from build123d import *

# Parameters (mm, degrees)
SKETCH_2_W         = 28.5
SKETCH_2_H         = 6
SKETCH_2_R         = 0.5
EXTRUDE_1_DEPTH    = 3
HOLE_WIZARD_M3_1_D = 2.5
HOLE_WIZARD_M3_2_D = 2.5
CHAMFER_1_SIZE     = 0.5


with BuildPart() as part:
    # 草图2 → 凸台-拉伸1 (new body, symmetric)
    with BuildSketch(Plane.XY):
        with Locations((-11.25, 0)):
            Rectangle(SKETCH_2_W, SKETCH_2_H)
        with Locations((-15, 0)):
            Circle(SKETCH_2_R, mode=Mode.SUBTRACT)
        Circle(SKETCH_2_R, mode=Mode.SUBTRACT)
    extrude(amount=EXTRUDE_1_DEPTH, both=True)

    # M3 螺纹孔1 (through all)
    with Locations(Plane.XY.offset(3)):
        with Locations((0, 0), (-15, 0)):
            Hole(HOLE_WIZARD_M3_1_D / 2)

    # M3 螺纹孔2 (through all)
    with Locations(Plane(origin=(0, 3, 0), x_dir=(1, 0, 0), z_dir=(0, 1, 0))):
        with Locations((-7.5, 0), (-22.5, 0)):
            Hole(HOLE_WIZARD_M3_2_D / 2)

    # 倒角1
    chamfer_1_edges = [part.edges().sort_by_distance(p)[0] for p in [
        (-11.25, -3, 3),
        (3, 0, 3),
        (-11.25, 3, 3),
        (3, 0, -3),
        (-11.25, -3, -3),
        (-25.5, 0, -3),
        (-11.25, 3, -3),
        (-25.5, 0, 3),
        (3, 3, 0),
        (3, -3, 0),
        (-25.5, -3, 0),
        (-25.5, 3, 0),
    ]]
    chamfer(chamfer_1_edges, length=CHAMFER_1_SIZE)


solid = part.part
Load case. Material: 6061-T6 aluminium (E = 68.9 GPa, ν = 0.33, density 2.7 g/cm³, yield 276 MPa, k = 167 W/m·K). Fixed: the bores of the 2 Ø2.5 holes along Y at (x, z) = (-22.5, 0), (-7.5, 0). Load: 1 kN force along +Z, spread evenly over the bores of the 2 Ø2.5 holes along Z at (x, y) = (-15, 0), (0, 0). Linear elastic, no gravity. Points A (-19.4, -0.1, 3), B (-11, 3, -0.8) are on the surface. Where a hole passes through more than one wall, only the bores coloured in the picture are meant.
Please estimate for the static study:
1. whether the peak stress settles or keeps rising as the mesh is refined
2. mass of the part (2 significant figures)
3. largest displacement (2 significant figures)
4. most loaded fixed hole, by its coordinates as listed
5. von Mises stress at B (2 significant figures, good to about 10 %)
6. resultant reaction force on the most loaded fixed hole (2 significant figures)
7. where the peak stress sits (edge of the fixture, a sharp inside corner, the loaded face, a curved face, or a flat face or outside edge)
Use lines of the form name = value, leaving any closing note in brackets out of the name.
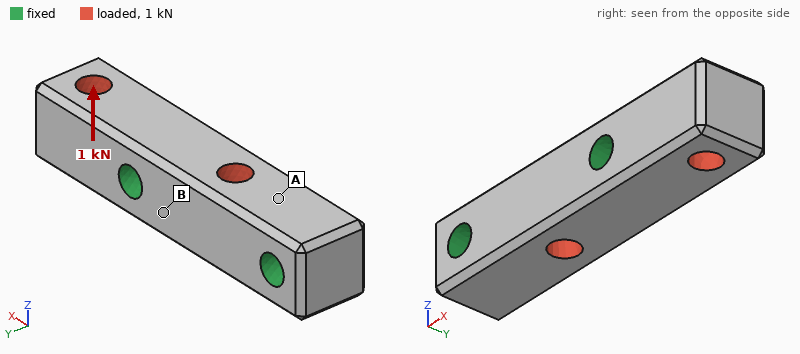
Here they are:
whether the peak stress settles or keeps rising as the mesh is refined = keeps rising
mass of the part = 2.4 g
largest displacement = 25 µm
most loaded fixed hole, by its coordinates as listed = (-7.5, 0)
von Mises stress at B = 22 MPa
resultant reaction force on the most loaded fixed hole = 810 N
where the peak stress sits = edge of the fixture
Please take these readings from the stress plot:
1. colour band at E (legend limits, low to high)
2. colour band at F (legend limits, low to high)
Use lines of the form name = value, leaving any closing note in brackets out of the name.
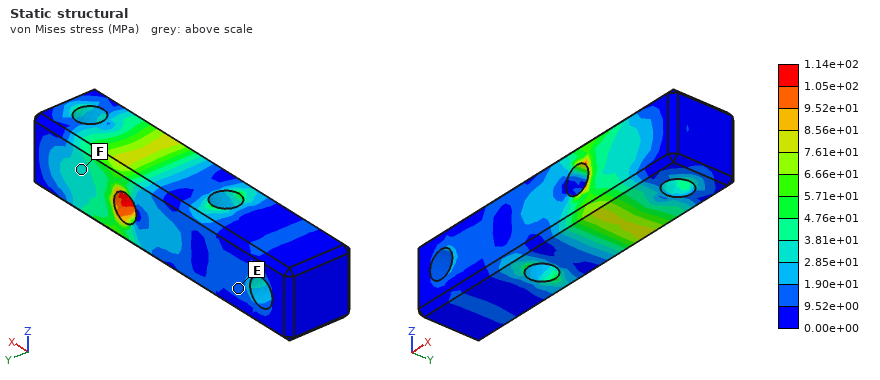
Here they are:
colour band at E = 9.52e+00 to 1.90e+01 MPa
colour band at F = 2.85e+01 to 3.81e+01 MPa
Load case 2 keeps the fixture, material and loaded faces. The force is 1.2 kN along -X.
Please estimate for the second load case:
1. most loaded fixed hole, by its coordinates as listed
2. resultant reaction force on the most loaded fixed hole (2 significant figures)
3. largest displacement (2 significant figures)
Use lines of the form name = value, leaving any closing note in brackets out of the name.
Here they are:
most loaded fixed hole, by its coordinates as listed = (-7.5, 0)
resultant reaction force on the most loaded fixed hole = 890 N
largest displacement = 3.0 µm
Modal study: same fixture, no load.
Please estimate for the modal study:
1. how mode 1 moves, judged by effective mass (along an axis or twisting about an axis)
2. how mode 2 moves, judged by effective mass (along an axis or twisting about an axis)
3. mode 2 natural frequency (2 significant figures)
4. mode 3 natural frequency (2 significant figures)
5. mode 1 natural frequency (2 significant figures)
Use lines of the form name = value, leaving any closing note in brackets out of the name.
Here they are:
how mode 1 moves, judged by effective mass = along Z
how mode 2 moves, judged by effective mass = along Y
mode 2 natural frequency = 40 kHz
mode 3 natural frequency = 73 kHz
mode 1 natural frequency = 35 kHz
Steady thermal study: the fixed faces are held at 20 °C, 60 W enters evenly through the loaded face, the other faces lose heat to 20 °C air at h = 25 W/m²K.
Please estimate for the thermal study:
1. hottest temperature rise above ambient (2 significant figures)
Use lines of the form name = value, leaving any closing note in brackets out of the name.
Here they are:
hottest temperature rise above ambient = 43 K
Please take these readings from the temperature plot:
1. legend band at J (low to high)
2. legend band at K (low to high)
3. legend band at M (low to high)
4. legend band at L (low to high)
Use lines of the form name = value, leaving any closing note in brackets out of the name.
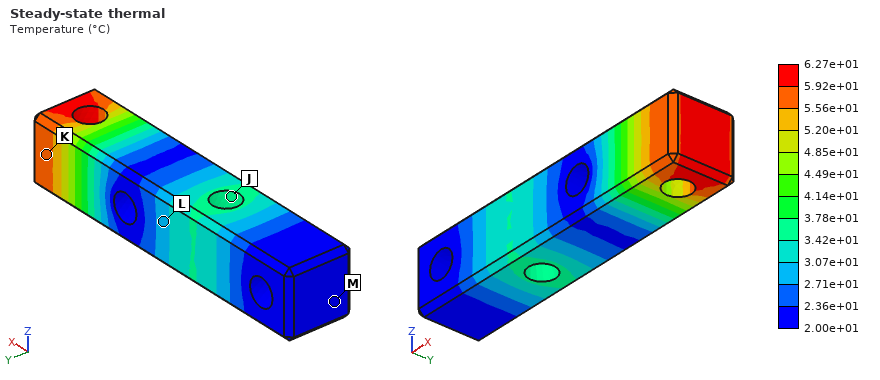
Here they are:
legend band at J = 3.42e+01 to 3.78e+01 °C
legend band at K = 5.56e+01 to 5.92e+01 °C
legend band at M = 2.00e+01 to 2.36e+01 °C
legend band at L = 2.71e+01 to 3.07e+01 °C
